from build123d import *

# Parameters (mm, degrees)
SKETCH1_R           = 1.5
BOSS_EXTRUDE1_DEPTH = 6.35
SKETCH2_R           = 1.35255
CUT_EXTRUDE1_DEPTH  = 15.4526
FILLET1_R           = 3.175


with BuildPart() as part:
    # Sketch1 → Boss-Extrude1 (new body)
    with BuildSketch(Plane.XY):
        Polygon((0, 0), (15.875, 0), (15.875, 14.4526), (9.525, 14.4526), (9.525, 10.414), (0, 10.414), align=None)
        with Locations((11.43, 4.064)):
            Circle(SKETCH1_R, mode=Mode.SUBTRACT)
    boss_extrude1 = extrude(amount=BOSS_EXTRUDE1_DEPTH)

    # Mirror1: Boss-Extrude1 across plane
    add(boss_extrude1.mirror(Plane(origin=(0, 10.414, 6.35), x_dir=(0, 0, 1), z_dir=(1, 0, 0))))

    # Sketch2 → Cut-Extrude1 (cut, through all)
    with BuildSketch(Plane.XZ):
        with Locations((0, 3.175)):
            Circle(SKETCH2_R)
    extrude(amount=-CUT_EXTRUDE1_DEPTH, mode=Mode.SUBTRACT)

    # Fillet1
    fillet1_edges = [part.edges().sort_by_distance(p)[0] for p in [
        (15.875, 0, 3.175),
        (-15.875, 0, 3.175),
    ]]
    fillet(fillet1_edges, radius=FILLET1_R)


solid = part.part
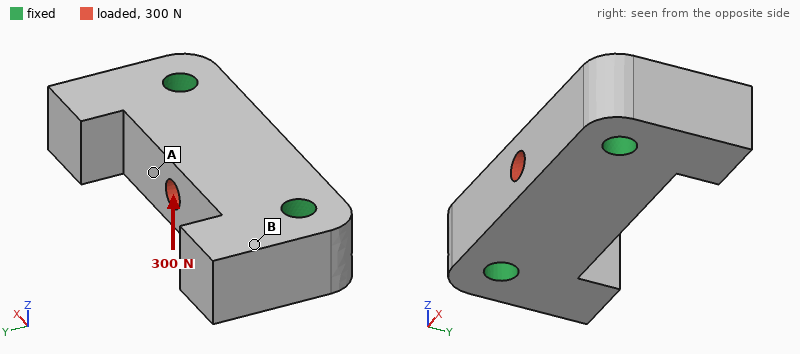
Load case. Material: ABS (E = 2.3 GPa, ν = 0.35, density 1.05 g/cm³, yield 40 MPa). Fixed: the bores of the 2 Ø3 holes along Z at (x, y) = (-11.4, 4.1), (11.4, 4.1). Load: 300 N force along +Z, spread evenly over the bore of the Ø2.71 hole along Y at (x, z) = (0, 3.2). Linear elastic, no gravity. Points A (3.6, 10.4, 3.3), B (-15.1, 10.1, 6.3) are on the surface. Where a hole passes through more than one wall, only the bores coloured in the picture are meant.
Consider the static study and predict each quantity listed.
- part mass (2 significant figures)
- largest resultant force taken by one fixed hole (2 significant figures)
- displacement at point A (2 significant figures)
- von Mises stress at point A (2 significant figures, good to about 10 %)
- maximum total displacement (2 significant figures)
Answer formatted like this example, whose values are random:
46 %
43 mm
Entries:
2.4 g
150 N
61 µm
6.7 MPa
81 µm
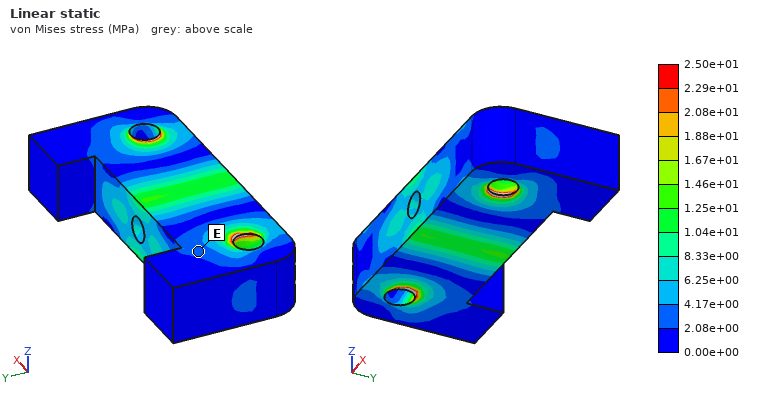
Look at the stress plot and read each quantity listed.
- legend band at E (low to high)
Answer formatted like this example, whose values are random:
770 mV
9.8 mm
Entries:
2.08e+00 to 4.17e+00 MPa
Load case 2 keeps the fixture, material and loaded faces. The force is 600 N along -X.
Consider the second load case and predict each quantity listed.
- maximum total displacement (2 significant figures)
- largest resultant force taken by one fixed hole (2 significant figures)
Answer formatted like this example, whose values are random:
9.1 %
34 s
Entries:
28 µm
300 N
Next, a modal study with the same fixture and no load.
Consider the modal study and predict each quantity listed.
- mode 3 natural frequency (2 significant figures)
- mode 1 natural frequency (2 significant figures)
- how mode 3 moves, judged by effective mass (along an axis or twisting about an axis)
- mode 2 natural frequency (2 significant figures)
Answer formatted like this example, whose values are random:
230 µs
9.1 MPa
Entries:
13 kHz
12 kHz
twisting about Y
12 kHz
